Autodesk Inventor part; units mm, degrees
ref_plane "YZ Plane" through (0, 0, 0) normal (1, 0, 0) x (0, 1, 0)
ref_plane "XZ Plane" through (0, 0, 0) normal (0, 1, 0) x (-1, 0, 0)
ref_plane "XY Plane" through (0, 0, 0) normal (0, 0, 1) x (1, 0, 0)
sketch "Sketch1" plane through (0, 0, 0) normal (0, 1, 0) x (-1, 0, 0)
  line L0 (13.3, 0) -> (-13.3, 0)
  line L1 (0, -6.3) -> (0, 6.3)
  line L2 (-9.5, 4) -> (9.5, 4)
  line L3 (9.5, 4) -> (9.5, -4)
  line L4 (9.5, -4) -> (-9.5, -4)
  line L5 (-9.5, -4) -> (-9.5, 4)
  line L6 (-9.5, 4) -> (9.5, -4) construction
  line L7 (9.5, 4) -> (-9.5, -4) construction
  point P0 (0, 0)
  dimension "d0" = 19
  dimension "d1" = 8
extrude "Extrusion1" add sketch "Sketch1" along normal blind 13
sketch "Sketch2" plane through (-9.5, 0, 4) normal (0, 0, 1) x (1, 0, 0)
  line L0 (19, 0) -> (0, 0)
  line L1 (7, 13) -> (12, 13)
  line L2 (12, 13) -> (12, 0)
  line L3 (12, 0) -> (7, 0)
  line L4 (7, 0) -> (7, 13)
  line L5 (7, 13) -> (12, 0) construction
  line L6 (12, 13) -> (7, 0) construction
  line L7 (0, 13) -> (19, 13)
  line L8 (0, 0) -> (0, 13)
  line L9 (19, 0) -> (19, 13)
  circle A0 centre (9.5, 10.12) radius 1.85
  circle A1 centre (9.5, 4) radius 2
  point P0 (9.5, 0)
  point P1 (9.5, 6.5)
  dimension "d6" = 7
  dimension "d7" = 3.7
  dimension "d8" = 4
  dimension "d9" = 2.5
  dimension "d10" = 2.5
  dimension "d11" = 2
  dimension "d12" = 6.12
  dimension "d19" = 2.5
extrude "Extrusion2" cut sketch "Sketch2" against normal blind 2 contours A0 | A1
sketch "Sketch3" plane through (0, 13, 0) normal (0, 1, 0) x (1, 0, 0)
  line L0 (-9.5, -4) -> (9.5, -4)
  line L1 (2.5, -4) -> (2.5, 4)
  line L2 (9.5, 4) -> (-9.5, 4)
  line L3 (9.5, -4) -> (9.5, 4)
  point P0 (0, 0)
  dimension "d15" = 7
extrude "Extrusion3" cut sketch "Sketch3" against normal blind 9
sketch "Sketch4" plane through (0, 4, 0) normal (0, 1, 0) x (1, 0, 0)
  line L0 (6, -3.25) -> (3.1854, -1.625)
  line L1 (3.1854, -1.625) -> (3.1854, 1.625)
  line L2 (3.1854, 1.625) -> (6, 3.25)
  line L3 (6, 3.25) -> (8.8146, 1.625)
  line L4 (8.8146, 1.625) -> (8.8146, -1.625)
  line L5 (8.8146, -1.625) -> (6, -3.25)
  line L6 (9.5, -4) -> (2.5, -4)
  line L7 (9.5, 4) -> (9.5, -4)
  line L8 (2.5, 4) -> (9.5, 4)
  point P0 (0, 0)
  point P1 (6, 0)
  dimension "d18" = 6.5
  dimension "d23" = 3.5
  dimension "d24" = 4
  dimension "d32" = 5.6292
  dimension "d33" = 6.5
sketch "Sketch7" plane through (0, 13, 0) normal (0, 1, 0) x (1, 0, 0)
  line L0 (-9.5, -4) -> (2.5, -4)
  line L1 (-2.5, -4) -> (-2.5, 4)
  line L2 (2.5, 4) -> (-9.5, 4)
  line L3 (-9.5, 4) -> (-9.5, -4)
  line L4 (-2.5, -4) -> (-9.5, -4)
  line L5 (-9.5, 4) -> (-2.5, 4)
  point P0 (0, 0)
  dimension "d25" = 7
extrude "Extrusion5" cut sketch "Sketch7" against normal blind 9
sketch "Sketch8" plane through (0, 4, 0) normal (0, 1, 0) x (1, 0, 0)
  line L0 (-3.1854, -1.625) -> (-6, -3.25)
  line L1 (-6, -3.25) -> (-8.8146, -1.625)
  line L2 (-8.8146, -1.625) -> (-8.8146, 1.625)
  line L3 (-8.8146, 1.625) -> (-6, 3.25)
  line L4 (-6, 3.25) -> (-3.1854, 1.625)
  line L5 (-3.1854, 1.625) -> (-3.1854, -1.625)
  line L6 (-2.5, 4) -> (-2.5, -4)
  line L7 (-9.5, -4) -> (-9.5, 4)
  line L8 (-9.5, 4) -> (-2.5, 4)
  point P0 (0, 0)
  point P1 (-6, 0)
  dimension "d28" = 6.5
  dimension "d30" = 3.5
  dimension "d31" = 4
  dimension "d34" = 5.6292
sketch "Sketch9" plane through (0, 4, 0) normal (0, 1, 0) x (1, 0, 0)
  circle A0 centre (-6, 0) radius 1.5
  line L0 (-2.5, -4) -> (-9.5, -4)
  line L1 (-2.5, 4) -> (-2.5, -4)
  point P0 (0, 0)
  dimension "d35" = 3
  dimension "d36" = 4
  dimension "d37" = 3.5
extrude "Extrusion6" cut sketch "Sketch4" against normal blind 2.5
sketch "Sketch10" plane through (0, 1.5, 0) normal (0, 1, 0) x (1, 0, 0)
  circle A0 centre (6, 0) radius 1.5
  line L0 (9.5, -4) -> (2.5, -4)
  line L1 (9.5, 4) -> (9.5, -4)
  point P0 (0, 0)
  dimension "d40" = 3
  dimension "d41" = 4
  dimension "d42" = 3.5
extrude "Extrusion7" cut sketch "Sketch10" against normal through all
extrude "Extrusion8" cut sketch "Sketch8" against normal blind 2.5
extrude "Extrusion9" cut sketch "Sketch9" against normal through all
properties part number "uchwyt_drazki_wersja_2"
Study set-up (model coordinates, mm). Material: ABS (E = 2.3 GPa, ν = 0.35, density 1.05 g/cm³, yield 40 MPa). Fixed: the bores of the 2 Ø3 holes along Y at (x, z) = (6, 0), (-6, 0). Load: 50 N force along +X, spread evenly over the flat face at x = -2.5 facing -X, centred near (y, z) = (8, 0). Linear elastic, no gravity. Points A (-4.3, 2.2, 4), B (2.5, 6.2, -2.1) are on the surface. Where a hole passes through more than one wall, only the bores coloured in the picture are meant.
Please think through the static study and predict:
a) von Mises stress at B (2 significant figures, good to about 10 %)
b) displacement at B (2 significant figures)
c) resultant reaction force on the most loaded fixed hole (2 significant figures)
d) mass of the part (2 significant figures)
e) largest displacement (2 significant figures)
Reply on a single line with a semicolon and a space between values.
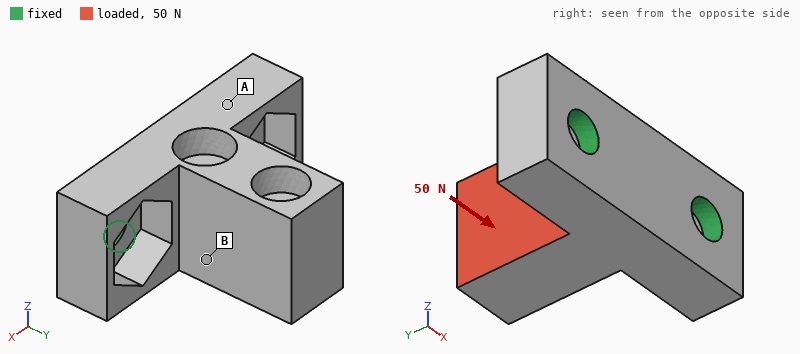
3.9 MPa; 0.037 mm; 46 N; 0.80 g; 0.11 mm
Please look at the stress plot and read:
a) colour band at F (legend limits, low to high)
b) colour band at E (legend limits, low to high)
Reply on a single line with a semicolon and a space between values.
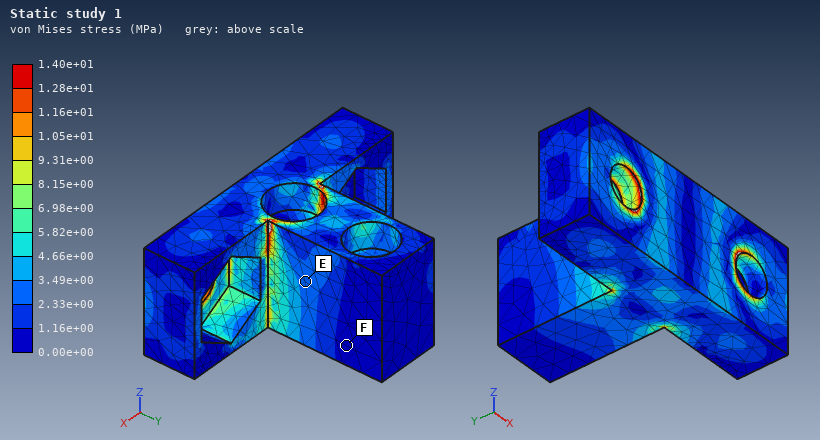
0.00e+00 to 1.16e+00 MPa; 2.33e+00 to 3.49e+00 MPa
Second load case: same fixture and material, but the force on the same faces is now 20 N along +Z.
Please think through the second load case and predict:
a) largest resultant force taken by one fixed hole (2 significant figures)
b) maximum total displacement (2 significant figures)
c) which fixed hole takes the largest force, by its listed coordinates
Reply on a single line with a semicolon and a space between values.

14 N; 0.12 mm; (-6, 0)
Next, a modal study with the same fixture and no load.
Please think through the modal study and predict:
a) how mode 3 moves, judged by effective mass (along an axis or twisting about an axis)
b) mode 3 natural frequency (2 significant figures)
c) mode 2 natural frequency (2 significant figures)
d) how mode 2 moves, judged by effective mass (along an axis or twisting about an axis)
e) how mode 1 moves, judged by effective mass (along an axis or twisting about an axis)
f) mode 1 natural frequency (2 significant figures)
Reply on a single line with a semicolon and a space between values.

along Y; 12 kHz; 7200 Hz; along X; along Z; 4100 Hz
